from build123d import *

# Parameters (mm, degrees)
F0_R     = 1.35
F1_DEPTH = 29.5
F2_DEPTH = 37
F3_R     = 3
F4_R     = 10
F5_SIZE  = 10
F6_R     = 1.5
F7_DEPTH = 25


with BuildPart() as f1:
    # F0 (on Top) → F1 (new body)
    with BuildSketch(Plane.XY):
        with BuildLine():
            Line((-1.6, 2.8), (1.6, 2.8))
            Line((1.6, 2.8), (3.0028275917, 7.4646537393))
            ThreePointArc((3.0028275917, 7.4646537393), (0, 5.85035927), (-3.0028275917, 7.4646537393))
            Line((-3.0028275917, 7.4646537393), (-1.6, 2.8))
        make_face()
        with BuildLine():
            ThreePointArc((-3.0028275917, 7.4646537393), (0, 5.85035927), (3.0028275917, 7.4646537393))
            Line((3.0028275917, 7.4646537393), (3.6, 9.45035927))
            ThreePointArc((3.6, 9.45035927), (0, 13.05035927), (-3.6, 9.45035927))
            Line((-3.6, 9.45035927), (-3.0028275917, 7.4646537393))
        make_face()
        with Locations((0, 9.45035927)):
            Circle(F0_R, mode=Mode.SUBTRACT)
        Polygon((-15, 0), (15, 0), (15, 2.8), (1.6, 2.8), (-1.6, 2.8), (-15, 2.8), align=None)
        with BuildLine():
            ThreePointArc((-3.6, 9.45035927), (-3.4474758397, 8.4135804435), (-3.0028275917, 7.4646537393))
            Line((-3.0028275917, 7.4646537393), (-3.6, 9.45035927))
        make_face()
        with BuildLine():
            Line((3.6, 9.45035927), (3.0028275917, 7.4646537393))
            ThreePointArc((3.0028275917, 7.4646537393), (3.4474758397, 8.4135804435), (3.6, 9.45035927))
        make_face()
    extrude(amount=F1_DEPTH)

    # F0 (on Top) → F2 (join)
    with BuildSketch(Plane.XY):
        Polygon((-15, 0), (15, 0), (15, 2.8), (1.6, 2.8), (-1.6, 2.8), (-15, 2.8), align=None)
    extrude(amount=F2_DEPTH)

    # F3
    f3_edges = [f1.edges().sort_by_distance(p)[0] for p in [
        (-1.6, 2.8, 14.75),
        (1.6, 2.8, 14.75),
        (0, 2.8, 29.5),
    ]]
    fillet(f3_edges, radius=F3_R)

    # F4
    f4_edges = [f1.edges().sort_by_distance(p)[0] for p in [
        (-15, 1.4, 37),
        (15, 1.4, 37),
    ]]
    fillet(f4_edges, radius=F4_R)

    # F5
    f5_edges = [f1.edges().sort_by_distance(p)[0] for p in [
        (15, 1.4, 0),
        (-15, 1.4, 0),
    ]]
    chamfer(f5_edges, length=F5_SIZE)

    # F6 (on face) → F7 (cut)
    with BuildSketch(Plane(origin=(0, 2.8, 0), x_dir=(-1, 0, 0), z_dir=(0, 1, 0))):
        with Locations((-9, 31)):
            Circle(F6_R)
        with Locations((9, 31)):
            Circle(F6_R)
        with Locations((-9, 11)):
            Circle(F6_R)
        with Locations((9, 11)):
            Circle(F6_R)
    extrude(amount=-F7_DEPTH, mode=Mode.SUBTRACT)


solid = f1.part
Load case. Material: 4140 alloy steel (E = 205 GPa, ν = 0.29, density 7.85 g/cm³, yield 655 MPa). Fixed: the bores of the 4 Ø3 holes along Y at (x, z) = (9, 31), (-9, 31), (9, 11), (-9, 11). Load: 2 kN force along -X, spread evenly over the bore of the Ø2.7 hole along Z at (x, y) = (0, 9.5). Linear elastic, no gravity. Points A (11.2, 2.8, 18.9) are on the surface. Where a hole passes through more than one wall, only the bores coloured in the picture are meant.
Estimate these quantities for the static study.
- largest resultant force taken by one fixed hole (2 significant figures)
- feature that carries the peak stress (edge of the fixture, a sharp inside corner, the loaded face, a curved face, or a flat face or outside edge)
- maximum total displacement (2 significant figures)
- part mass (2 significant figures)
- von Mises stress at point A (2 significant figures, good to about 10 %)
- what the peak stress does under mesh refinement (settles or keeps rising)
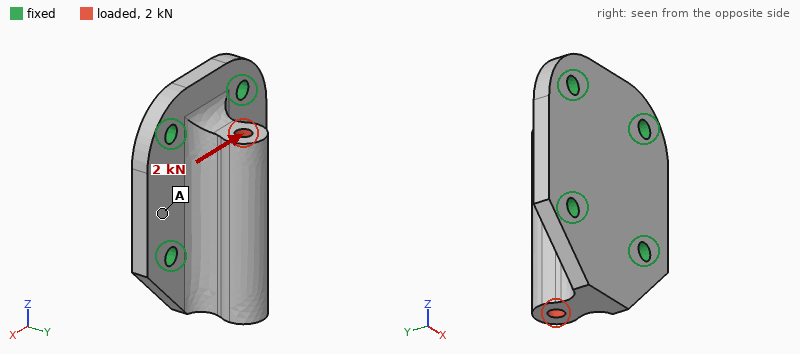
1.0 kN
edge of the fixture
14 µm
34 g
13 MPa
keeps rising
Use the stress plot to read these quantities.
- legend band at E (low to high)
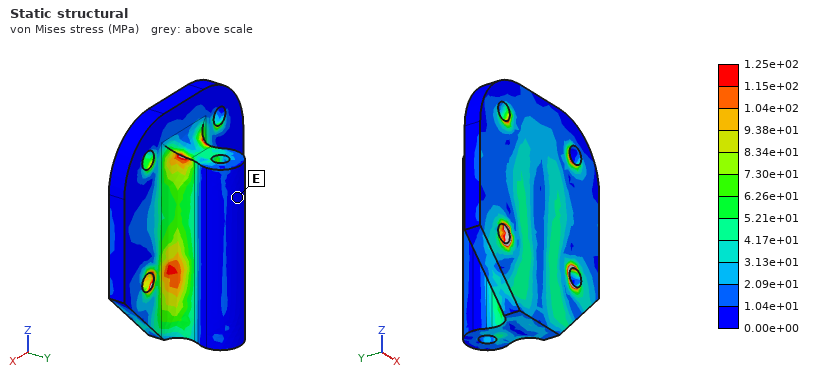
0.00e+00 to 1.04e+01 MPa
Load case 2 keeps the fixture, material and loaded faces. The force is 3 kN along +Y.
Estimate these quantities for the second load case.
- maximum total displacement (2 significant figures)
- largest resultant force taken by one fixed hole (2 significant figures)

12 µm
1.3 kN
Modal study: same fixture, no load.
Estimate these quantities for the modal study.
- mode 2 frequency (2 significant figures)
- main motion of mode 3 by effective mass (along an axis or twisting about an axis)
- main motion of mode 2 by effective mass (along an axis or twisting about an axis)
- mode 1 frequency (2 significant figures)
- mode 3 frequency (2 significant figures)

23 kHz
along Y
along X
19 kHz
26 kHz
